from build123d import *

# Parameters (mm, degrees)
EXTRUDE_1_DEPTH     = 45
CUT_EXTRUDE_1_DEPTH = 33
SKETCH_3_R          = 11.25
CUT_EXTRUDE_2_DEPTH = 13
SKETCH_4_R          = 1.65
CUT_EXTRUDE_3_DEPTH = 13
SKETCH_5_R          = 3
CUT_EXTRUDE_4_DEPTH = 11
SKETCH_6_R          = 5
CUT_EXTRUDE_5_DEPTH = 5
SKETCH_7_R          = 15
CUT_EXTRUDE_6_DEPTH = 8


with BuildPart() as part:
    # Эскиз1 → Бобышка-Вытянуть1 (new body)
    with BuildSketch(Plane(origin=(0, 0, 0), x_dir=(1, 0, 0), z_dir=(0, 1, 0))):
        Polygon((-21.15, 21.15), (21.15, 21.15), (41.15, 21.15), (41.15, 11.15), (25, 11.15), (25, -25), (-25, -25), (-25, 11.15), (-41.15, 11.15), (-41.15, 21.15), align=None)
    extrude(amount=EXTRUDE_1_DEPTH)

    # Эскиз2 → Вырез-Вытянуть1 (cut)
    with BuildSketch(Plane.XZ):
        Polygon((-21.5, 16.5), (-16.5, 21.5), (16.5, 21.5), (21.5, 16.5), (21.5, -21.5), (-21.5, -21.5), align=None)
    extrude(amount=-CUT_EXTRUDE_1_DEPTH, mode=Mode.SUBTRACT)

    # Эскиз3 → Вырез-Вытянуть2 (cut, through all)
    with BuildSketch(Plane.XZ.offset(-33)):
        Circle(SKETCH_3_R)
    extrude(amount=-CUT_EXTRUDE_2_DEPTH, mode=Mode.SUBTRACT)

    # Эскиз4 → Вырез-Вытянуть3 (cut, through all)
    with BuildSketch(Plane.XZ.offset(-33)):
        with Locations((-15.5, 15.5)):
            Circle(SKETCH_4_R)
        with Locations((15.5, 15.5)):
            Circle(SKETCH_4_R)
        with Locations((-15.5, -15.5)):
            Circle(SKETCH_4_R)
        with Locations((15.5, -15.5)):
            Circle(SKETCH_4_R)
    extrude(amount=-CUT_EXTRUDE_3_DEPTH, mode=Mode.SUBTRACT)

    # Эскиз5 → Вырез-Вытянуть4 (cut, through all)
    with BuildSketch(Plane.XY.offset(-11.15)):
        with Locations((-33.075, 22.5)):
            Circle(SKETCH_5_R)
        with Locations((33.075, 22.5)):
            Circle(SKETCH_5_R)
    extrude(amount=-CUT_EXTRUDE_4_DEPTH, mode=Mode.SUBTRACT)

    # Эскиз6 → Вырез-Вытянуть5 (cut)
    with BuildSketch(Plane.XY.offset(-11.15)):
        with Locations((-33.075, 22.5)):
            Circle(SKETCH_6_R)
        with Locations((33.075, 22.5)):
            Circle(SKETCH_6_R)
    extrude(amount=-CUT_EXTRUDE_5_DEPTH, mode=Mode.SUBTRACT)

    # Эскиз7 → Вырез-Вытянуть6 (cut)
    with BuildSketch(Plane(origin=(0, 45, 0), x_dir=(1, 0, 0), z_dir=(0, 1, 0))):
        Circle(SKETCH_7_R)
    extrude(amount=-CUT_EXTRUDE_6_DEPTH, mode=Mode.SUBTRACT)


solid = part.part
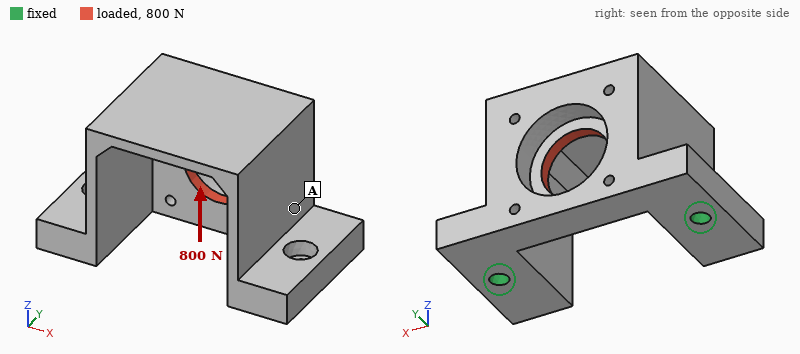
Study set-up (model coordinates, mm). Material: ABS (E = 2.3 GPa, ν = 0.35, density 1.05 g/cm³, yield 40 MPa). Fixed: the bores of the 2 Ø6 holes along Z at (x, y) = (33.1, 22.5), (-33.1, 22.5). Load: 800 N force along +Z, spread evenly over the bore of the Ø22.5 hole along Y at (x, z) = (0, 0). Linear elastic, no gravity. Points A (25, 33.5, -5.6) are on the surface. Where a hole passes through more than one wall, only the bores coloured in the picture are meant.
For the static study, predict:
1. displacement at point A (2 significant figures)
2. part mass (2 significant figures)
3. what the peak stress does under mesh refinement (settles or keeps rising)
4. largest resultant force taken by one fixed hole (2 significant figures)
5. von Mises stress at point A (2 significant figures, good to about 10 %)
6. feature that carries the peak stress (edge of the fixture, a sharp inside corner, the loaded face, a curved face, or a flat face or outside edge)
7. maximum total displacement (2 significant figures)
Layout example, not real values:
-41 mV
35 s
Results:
0.38 mm
52 g
keeps rising
410 N
6.4 MPa
edge of the fixture
0.98 mm
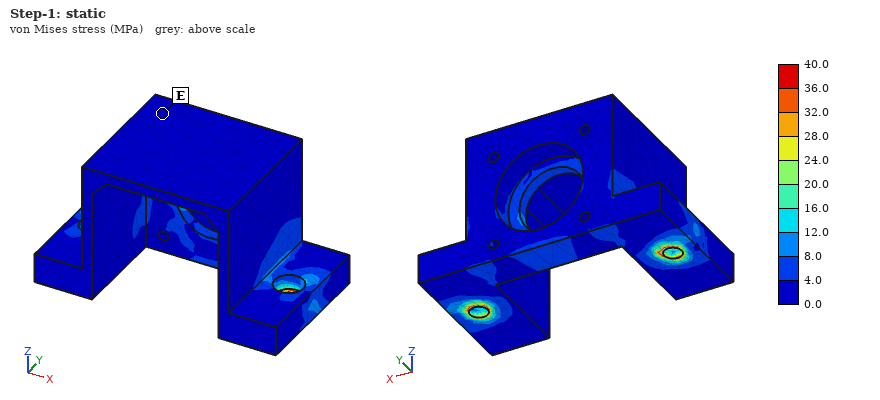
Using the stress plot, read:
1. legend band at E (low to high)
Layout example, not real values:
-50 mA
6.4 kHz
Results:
0.0 to 4.0 MPa
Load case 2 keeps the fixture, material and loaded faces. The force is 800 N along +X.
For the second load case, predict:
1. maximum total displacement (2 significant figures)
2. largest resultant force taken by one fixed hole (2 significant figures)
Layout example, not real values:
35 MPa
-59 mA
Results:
0.51 mm
460 N
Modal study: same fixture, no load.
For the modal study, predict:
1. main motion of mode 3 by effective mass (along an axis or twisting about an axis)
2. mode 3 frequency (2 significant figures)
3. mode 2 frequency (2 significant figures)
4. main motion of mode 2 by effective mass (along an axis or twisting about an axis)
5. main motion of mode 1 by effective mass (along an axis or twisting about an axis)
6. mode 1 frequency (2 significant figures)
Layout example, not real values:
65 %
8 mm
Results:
along X
1900 Hz
870 Hz
along X
along Y
550 Hz
